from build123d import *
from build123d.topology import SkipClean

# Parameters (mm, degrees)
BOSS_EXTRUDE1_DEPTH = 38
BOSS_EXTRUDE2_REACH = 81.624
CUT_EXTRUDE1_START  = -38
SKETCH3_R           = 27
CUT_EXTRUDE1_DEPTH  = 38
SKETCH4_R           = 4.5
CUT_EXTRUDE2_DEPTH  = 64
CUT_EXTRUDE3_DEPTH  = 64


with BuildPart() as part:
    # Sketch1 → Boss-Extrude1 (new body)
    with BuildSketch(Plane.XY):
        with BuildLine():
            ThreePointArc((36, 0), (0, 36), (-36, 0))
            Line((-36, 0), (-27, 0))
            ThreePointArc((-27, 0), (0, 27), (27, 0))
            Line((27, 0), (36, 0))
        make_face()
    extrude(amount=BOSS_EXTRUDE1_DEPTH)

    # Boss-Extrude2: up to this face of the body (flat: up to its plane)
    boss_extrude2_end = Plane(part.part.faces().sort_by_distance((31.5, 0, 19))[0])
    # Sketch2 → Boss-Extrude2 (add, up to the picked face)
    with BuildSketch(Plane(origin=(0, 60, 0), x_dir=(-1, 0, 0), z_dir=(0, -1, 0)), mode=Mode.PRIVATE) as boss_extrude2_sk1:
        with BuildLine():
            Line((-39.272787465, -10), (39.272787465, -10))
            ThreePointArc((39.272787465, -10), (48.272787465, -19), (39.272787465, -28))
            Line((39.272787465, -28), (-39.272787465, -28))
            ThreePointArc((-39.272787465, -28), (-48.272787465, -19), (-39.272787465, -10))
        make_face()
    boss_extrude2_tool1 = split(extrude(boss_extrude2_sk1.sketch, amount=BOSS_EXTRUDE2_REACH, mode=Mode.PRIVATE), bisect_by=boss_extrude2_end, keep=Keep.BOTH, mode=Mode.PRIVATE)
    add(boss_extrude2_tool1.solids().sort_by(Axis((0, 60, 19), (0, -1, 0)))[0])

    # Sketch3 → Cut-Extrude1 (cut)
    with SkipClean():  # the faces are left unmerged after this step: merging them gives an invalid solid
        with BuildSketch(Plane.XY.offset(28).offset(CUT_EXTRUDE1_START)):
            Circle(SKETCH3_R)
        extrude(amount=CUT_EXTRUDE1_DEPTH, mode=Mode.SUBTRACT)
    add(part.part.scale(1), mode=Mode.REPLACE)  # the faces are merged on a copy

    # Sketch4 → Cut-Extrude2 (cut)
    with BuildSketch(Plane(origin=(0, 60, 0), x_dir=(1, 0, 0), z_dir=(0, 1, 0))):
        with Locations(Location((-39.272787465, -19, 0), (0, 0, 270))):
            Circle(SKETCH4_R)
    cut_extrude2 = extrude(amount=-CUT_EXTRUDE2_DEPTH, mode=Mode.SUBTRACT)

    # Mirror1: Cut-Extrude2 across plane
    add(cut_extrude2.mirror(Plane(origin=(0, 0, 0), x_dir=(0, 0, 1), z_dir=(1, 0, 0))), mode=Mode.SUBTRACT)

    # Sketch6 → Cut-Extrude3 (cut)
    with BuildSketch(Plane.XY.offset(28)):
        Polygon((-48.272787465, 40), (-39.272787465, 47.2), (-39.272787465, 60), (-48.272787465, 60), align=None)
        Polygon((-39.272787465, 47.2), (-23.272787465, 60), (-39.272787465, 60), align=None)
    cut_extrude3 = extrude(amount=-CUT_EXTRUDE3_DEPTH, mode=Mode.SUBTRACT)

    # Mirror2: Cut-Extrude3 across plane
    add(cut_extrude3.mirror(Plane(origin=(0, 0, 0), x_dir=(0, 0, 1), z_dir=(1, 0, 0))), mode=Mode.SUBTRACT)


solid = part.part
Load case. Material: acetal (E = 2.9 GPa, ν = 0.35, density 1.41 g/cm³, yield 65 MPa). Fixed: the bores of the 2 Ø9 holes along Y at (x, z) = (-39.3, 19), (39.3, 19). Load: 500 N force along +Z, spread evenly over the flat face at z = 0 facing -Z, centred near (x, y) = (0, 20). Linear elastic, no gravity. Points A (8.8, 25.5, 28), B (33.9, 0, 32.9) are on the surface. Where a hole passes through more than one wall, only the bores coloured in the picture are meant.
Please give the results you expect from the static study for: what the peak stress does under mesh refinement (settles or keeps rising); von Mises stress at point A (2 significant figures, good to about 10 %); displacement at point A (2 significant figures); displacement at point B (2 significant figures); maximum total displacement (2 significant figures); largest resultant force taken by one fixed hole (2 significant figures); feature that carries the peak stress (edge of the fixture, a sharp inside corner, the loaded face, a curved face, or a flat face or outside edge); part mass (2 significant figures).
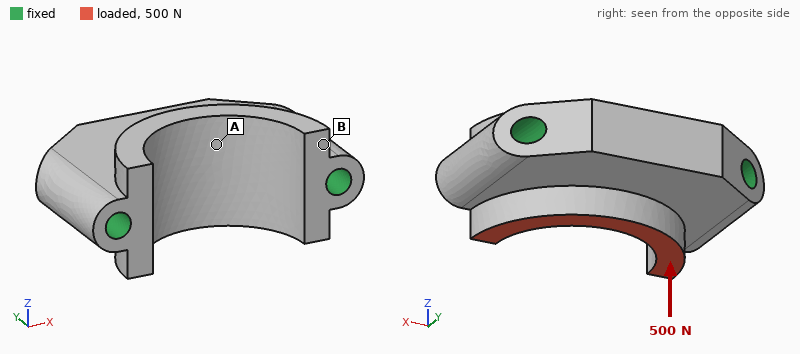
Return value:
keeps rising
0.49 MPa
10 µm
3.7 µm
14 µm
250 N
edge of the fixture
120 g
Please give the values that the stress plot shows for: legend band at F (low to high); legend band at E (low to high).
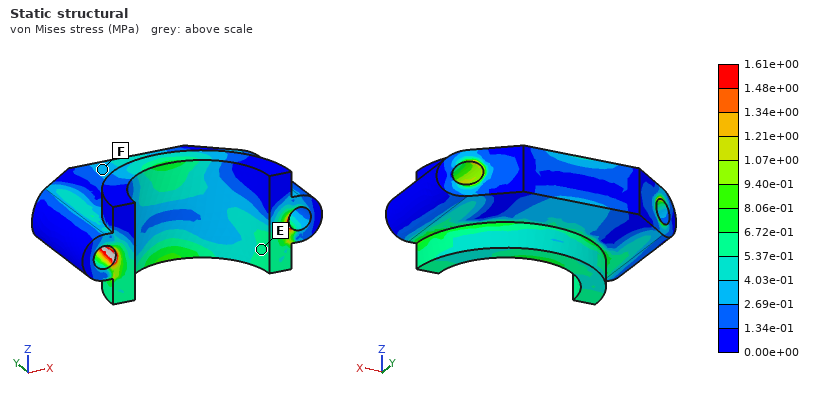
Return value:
2.69e-01 to 4.03e-01 MPa
5.37e-01 to 6.72e-01 MPa
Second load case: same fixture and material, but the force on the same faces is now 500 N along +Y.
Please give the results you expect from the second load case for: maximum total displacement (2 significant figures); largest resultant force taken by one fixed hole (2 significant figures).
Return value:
36 µm
260 N
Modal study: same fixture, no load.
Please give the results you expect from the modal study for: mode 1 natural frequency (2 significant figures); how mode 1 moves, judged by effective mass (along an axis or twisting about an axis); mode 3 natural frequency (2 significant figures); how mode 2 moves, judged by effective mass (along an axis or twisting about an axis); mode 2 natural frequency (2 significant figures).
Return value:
3100 Hz
along Z
5400 Hz
along Y
5000 Hz
